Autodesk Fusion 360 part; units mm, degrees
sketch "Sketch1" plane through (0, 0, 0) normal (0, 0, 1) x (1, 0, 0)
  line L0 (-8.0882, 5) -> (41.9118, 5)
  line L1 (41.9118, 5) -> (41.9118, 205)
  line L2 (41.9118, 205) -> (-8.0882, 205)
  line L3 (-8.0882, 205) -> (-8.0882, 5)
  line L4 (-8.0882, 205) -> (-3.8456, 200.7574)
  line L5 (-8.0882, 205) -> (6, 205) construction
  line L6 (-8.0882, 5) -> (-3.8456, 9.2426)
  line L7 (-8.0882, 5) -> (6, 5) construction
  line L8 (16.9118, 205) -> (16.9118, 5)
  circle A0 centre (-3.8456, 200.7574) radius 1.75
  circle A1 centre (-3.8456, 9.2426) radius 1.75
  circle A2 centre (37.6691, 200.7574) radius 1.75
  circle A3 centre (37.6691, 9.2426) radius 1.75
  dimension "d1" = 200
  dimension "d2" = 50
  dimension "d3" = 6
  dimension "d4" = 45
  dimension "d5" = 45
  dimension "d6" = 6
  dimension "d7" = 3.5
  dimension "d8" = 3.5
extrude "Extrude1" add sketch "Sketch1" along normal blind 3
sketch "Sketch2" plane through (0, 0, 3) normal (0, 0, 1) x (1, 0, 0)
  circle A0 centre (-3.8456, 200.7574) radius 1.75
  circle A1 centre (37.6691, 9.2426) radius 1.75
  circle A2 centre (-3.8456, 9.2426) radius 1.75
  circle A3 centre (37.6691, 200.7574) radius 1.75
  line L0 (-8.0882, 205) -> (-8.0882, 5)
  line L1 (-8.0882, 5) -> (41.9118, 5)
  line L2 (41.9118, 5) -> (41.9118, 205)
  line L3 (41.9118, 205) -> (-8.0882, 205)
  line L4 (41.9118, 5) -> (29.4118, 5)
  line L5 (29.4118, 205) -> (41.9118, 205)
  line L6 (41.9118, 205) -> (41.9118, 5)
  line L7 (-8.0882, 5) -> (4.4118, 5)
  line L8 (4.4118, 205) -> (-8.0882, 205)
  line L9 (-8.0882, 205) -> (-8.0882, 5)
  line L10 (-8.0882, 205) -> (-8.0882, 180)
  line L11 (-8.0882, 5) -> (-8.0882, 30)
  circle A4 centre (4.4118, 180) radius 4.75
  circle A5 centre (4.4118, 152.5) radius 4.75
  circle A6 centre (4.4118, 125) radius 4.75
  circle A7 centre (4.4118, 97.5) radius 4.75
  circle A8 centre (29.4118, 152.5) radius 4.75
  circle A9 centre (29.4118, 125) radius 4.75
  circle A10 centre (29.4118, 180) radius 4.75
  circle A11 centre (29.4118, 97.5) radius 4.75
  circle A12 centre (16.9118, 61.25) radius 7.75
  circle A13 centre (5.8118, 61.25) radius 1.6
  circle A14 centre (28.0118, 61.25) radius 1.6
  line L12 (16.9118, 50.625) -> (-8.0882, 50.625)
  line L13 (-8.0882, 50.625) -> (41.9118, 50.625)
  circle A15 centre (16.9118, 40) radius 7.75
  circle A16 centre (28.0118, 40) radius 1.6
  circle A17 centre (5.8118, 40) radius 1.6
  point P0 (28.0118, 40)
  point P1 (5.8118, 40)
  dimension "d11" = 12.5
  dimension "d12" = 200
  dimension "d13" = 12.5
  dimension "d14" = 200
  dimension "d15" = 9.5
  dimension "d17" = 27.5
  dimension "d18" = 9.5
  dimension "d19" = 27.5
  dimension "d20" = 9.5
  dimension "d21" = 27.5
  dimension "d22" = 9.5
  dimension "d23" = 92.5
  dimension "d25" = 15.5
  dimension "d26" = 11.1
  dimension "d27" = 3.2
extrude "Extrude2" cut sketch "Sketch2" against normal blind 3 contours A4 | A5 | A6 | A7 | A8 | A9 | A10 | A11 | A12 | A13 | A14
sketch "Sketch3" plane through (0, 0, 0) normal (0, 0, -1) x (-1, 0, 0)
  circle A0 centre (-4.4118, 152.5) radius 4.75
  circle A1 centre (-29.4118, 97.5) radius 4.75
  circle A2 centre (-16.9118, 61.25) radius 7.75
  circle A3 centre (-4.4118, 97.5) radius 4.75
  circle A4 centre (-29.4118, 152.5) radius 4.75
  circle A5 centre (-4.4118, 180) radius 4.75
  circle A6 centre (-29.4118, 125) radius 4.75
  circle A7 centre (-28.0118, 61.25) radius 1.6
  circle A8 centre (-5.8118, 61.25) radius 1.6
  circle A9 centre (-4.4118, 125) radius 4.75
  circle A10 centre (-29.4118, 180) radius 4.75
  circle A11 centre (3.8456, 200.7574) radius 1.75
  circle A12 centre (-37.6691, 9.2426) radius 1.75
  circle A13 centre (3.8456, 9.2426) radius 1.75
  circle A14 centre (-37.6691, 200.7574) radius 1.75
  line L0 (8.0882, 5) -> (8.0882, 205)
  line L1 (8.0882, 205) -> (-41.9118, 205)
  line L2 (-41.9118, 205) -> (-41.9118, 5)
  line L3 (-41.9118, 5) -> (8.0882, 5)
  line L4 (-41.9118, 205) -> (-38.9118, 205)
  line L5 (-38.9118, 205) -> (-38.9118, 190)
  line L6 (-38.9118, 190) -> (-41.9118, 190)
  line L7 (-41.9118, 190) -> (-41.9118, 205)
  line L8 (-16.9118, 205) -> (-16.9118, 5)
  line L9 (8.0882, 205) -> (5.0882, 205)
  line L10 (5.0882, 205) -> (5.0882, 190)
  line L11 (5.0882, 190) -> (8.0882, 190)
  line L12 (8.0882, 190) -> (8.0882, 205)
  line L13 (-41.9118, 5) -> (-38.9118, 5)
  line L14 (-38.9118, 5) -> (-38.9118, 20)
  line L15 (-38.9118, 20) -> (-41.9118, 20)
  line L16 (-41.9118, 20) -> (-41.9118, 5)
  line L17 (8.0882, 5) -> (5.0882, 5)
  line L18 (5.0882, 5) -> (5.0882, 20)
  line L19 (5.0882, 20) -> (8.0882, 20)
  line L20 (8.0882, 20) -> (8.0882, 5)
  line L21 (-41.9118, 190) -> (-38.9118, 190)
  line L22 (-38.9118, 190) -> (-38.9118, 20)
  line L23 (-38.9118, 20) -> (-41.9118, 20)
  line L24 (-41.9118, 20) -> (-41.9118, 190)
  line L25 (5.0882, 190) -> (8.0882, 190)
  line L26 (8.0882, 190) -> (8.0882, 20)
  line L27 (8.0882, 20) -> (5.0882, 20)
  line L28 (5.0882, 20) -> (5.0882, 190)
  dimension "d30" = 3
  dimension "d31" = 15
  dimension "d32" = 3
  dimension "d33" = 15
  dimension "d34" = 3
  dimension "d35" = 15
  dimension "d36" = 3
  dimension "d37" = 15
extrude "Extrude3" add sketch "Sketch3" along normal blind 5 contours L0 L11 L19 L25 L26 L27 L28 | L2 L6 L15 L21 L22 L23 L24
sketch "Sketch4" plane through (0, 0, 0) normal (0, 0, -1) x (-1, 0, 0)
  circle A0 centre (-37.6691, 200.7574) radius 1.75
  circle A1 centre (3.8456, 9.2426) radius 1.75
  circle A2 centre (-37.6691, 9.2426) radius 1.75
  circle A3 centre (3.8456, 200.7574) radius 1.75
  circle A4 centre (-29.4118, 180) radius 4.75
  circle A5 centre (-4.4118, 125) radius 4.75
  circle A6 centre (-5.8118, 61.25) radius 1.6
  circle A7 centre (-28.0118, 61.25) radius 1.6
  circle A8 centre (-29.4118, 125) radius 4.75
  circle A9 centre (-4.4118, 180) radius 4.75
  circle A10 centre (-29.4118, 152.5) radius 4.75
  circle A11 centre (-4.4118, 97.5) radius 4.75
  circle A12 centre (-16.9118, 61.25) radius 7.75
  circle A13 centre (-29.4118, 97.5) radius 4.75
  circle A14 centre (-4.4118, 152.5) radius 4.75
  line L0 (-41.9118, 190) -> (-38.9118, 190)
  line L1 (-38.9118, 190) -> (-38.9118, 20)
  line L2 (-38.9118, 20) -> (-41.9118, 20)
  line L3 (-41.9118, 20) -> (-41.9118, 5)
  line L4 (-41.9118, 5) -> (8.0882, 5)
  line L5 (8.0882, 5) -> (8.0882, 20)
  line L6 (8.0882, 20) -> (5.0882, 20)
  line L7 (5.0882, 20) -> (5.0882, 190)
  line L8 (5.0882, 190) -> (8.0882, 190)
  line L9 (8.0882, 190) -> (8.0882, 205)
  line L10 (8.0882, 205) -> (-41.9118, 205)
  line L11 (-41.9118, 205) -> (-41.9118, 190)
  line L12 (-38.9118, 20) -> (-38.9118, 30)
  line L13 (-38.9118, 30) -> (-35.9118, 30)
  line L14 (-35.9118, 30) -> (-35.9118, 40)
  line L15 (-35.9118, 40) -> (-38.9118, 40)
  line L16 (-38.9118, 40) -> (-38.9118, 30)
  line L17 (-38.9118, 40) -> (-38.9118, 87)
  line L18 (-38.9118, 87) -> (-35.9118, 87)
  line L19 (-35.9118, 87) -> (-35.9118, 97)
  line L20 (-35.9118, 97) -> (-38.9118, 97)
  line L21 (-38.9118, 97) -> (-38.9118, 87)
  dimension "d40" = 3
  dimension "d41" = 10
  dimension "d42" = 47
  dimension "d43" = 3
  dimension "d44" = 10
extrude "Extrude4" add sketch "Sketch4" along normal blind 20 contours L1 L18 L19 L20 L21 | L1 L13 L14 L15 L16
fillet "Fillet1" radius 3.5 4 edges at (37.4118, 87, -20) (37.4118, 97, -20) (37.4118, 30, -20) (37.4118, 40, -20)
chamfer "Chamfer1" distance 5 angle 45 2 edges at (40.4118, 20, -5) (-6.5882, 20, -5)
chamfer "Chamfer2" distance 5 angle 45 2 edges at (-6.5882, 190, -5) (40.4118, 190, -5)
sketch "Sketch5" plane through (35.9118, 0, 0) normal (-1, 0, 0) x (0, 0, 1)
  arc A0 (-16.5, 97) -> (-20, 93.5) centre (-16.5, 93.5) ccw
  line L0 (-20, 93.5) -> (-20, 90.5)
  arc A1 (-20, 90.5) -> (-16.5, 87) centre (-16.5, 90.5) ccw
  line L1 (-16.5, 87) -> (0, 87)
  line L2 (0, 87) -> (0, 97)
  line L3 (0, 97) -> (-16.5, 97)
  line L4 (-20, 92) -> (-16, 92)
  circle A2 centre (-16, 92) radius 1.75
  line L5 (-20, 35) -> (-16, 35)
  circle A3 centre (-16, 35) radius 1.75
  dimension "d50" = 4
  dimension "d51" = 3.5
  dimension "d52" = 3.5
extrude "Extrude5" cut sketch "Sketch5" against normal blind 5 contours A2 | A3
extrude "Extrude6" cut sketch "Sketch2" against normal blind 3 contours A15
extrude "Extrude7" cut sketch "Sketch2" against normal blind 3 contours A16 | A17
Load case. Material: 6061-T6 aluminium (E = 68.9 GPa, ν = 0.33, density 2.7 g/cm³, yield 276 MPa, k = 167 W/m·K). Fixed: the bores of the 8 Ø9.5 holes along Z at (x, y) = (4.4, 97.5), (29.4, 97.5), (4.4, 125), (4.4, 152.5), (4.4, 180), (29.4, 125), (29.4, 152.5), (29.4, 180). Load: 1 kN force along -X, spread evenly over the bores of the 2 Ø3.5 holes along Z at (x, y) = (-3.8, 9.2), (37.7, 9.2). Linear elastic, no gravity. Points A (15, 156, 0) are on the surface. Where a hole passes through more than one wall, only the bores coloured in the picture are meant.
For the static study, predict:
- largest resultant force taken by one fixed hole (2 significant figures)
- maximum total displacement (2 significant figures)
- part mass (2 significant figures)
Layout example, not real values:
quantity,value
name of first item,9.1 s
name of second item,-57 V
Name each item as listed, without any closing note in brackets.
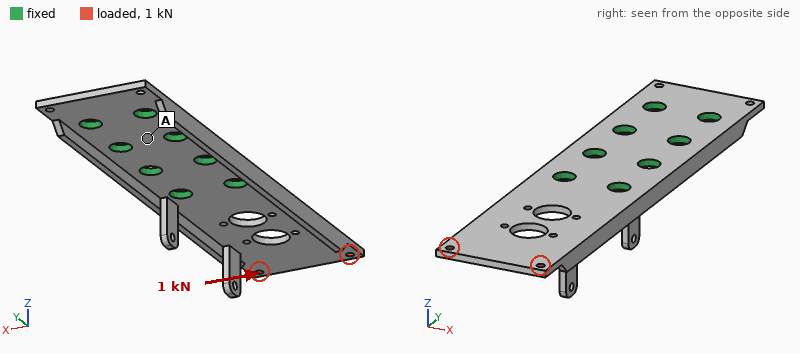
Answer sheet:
quantity,value
largest resultant force taken by one fixed hole,2.2 kN
maximum total displacement,0.21 mm
part mass,89 g
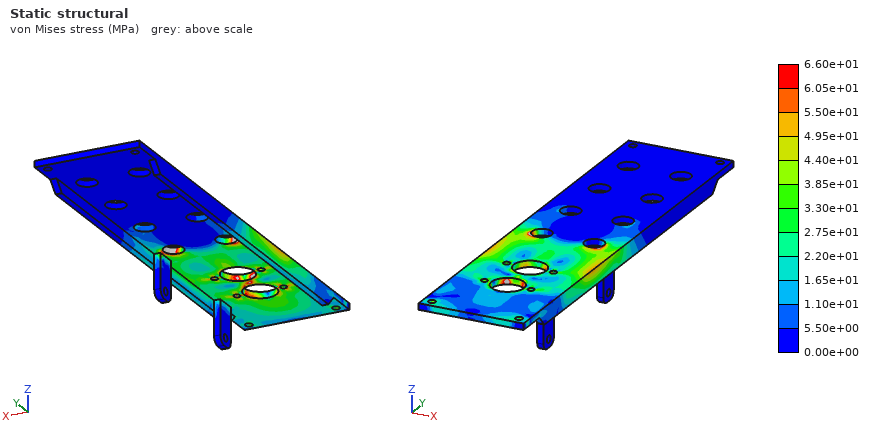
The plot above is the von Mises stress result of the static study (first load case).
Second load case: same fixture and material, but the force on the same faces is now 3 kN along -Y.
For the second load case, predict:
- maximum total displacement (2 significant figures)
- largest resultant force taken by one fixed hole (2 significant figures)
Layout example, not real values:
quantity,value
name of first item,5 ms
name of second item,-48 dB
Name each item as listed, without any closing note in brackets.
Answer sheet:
quantity,value
maximum total displacement,0.25 mm
largest resultant force taken by one fixed hole,1.3 kN
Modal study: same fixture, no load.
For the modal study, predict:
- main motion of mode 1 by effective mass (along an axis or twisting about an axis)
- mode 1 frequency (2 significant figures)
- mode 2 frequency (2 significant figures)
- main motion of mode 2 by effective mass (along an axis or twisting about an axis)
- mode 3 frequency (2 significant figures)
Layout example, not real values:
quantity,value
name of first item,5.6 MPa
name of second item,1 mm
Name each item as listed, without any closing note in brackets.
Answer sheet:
quantity,value
main motion of mode 1 by effective mass,along Z
mode 1 frequency,580 Hz
mode 2 frequency,1200 Hz
main motion of mode 2 by effective mass,twisting about Y
mode 3 frequency,3100 Hz
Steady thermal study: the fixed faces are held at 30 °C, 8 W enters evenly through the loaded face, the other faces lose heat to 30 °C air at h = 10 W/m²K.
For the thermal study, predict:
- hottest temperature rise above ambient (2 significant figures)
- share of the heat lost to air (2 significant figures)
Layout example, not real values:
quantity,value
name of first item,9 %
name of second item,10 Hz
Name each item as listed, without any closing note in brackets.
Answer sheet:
quantity,value
hottest temperature rise above ambient,28 K
share of the heat lost to air,17 %
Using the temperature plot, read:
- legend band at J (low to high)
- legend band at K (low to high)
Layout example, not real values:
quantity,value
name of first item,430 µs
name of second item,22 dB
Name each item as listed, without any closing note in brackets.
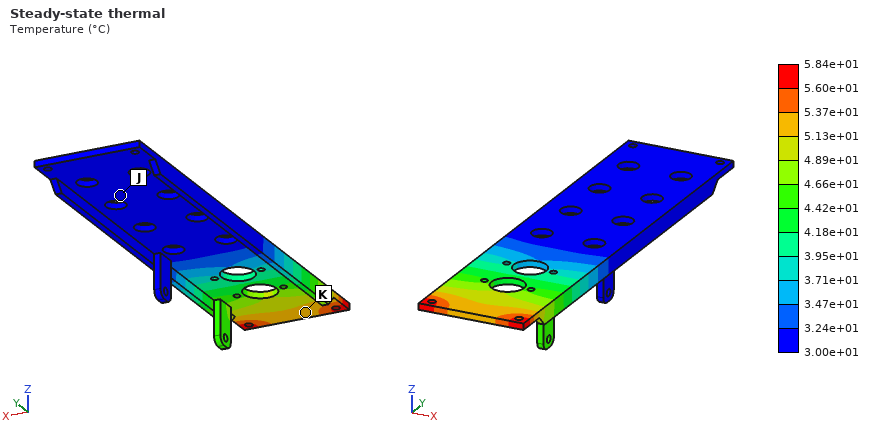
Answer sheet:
quantity,value
legend band at J,3.00e+01 to 3.24e+01 °C
legend band at K,5.13e+01 to 5.37e+01 °C
